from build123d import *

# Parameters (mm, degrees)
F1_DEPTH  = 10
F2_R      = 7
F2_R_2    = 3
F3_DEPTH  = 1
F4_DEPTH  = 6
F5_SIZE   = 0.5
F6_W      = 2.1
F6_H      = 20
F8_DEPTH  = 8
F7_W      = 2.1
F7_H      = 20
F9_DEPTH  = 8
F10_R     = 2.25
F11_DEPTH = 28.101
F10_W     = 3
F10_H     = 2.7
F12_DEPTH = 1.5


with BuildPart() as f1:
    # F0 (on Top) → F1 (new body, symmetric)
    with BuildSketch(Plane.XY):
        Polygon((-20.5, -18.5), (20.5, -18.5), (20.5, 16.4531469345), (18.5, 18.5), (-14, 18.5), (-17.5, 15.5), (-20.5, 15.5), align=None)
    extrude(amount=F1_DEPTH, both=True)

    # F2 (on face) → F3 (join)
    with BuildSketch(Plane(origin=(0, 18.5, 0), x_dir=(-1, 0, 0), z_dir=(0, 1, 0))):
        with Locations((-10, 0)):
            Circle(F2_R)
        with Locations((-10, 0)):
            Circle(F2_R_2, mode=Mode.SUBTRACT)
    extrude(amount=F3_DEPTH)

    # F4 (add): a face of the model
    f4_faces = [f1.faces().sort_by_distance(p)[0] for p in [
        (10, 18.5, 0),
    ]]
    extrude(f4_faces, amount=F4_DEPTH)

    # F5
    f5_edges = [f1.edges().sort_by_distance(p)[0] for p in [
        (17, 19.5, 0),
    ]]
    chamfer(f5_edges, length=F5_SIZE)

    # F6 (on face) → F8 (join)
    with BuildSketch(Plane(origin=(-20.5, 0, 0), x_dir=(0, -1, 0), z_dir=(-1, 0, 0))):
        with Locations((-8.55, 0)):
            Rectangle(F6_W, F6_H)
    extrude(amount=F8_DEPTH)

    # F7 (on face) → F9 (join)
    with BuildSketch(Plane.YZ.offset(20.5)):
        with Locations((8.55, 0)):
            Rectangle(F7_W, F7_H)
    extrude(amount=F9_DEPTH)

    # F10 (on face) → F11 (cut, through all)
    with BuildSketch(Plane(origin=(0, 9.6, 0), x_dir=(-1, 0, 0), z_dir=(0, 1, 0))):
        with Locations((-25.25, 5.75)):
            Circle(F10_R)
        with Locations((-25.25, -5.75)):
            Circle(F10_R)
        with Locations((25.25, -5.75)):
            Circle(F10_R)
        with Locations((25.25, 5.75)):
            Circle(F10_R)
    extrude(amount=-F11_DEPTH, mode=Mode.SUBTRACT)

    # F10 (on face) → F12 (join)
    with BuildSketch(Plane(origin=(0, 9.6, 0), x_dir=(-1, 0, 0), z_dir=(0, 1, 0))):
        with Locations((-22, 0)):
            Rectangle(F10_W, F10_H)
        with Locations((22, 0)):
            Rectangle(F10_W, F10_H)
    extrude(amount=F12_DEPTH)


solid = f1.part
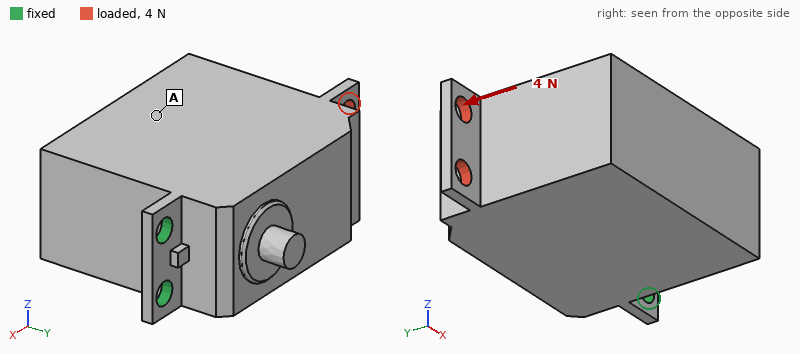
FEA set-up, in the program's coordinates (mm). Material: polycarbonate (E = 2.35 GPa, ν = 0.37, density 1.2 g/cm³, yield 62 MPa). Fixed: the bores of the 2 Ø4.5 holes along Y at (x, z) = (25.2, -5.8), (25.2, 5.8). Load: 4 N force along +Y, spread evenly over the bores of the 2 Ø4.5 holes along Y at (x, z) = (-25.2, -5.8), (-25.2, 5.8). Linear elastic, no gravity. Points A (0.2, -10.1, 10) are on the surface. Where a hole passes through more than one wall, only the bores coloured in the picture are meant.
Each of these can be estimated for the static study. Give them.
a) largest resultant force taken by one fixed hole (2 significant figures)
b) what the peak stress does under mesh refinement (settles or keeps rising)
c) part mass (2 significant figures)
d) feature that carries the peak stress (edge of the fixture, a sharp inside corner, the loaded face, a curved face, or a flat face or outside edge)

2.3 N
keeps rising
37 g
edge of the fixture
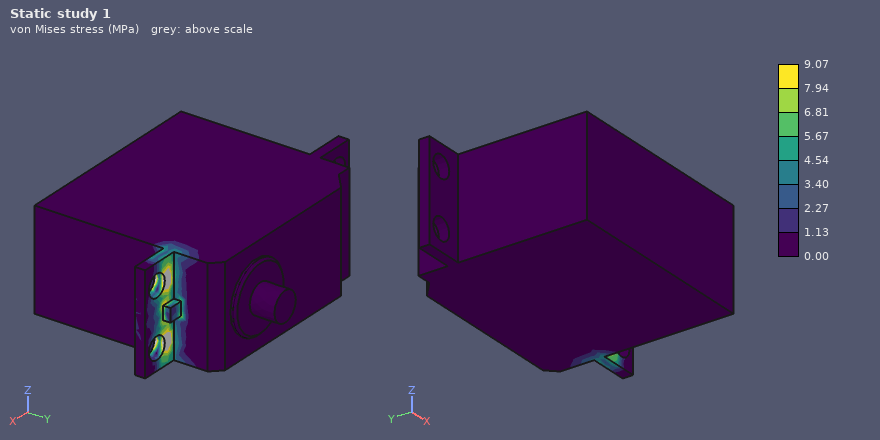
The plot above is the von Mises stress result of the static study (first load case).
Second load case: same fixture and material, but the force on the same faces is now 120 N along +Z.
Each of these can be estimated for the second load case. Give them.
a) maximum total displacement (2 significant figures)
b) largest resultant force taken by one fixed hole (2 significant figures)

0.72 mm
450 N
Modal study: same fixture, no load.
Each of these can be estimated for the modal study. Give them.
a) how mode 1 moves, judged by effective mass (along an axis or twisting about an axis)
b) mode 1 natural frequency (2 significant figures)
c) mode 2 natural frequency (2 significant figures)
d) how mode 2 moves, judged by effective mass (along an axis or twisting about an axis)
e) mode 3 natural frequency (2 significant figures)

along Y
100 Hz
550 Hz
along Z
950 Hz
